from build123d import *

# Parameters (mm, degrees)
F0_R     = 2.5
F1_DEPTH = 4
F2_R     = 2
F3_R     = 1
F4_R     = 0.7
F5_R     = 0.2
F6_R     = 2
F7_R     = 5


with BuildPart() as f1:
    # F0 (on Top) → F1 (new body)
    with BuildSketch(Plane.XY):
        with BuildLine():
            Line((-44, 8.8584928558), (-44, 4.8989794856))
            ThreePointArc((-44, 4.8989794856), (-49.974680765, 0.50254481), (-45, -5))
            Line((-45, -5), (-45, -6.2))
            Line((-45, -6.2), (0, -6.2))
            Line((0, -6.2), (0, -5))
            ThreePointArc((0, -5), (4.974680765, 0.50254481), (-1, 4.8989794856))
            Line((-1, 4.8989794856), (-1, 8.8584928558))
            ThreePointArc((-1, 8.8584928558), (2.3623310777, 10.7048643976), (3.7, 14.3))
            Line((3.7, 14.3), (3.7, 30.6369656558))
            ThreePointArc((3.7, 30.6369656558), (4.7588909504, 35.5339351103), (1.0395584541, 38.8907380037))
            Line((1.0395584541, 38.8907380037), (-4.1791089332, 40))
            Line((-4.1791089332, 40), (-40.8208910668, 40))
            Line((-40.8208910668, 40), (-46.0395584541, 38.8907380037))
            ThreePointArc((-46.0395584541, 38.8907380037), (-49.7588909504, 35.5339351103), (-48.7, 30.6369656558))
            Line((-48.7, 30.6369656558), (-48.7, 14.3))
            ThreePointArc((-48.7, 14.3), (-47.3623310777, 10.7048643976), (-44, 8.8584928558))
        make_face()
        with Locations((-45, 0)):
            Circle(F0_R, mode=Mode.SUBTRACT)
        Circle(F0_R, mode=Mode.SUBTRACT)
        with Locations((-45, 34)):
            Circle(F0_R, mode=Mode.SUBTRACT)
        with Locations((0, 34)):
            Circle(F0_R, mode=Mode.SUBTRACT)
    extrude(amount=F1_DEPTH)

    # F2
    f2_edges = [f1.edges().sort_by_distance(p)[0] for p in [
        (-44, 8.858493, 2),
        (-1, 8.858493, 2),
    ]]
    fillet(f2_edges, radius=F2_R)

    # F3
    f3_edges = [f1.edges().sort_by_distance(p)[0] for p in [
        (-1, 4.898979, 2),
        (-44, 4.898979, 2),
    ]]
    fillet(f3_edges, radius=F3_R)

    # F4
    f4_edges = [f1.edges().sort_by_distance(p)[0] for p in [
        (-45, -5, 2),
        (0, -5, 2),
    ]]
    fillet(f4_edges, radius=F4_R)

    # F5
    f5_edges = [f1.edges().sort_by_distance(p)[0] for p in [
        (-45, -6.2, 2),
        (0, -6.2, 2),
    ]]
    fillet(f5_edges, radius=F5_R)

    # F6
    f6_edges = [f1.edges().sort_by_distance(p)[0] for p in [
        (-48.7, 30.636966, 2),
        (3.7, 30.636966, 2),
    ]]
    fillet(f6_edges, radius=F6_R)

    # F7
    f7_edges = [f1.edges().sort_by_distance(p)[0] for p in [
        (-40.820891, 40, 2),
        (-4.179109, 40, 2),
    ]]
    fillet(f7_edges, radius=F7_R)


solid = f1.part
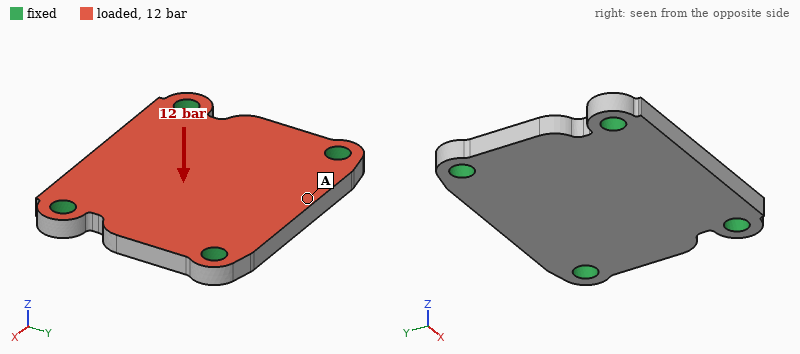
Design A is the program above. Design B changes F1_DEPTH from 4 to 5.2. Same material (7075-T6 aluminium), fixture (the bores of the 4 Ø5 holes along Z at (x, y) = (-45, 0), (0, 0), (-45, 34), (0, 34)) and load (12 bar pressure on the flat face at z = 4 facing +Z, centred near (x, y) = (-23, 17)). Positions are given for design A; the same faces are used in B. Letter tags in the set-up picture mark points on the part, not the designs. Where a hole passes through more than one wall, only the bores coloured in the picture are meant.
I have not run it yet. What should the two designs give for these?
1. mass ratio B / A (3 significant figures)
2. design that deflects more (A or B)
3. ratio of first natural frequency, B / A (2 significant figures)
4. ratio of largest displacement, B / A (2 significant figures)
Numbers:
1.30
A
1.2
0.50
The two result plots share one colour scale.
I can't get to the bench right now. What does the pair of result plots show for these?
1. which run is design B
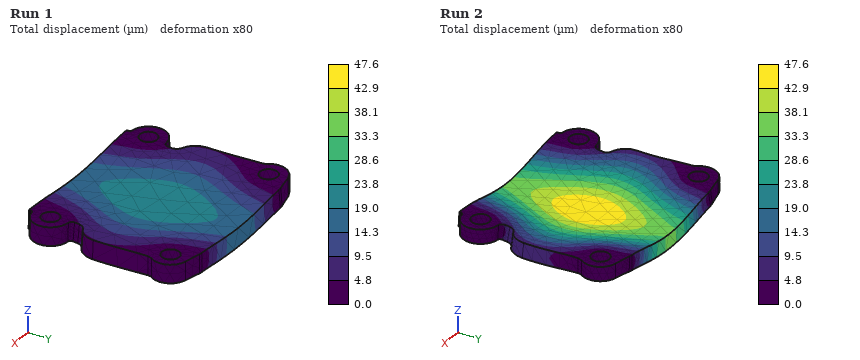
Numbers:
Run 1
